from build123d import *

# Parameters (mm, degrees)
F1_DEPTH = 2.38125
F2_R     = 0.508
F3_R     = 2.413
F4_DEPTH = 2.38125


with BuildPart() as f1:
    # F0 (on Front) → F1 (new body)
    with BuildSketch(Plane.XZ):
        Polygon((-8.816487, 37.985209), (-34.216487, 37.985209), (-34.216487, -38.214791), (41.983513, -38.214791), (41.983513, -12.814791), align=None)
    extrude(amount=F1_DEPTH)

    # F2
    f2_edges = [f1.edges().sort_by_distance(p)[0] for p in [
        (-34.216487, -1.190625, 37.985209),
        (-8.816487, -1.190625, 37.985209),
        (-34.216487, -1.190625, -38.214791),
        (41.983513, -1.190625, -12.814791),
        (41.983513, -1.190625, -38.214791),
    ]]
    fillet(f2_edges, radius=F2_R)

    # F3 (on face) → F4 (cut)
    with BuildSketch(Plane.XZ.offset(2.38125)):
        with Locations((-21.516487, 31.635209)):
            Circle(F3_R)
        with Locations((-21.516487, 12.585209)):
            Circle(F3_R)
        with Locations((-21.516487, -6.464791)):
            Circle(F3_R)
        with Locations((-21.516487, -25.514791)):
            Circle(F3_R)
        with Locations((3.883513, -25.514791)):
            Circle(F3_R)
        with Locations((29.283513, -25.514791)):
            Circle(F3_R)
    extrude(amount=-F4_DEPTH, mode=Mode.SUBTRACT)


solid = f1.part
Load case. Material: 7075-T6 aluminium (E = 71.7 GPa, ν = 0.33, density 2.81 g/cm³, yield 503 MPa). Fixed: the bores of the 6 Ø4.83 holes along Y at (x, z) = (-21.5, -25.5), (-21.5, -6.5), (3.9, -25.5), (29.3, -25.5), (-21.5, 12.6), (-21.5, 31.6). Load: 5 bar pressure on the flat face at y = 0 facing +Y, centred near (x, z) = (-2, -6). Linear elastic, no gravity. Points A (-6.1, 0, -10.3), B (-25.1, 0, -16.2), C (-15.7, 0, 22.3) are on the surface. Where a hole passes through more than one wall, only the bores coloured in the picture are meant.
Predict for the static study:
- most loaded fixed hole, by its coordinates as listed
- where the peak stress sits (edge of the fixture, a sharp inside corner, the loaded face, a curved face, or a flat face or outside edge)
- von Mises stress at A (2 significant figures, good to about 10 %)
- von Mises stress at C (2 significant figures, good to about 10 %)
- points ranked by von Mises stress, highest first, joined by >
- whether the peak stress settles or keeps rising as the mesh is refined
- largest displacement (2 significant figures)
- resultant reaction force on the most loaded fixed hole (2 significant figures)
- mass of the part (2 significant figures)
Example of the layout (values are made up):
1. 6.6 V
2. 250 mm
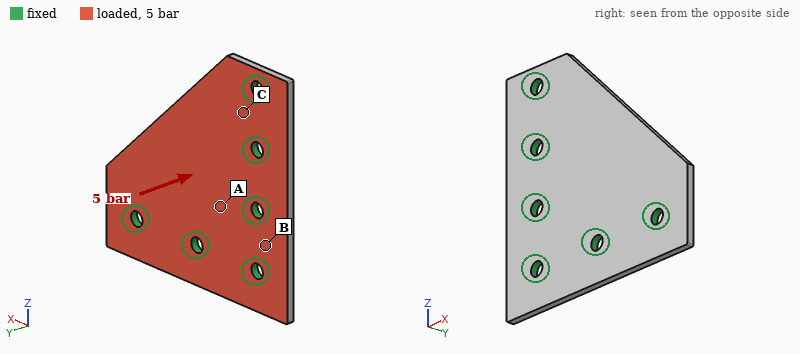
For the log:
1. (29.3, -25.5)
2. edge of the fixture
3. 55 MPa
4. 90 MPa
5. C > A > B
6. keeps rising
7. 0.43 mm
8. 510 N
9. 29 g
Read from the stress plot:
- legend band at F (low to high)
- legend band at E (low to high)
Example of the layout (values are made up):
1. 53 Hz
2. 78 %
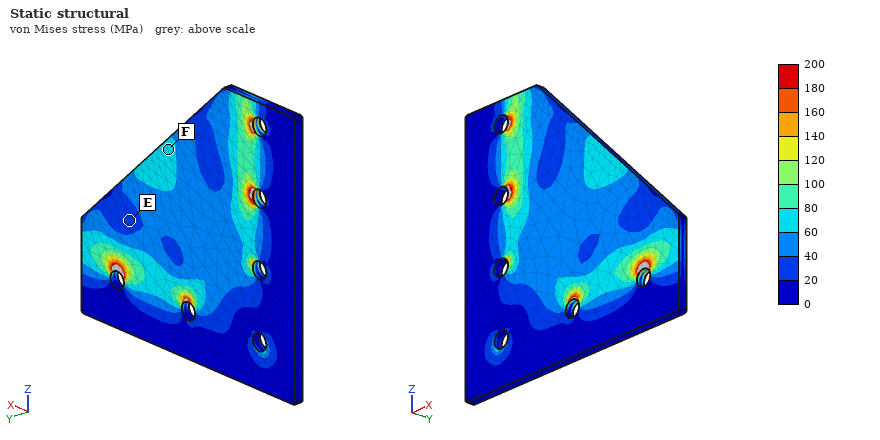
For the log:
1. 60 to 80 MPa
2. 20 to 40 MPa
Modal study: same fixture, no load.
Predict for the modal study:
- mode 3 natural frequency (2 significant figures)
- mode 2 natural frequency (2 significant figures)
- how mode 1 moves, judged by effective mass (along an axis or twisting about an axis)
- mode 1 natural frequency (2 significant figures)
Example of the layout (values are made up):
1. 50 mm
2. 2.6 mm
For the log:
1. 8500 Hz
2. 6100 Hz
3. along Y
4. 2900 Hz
